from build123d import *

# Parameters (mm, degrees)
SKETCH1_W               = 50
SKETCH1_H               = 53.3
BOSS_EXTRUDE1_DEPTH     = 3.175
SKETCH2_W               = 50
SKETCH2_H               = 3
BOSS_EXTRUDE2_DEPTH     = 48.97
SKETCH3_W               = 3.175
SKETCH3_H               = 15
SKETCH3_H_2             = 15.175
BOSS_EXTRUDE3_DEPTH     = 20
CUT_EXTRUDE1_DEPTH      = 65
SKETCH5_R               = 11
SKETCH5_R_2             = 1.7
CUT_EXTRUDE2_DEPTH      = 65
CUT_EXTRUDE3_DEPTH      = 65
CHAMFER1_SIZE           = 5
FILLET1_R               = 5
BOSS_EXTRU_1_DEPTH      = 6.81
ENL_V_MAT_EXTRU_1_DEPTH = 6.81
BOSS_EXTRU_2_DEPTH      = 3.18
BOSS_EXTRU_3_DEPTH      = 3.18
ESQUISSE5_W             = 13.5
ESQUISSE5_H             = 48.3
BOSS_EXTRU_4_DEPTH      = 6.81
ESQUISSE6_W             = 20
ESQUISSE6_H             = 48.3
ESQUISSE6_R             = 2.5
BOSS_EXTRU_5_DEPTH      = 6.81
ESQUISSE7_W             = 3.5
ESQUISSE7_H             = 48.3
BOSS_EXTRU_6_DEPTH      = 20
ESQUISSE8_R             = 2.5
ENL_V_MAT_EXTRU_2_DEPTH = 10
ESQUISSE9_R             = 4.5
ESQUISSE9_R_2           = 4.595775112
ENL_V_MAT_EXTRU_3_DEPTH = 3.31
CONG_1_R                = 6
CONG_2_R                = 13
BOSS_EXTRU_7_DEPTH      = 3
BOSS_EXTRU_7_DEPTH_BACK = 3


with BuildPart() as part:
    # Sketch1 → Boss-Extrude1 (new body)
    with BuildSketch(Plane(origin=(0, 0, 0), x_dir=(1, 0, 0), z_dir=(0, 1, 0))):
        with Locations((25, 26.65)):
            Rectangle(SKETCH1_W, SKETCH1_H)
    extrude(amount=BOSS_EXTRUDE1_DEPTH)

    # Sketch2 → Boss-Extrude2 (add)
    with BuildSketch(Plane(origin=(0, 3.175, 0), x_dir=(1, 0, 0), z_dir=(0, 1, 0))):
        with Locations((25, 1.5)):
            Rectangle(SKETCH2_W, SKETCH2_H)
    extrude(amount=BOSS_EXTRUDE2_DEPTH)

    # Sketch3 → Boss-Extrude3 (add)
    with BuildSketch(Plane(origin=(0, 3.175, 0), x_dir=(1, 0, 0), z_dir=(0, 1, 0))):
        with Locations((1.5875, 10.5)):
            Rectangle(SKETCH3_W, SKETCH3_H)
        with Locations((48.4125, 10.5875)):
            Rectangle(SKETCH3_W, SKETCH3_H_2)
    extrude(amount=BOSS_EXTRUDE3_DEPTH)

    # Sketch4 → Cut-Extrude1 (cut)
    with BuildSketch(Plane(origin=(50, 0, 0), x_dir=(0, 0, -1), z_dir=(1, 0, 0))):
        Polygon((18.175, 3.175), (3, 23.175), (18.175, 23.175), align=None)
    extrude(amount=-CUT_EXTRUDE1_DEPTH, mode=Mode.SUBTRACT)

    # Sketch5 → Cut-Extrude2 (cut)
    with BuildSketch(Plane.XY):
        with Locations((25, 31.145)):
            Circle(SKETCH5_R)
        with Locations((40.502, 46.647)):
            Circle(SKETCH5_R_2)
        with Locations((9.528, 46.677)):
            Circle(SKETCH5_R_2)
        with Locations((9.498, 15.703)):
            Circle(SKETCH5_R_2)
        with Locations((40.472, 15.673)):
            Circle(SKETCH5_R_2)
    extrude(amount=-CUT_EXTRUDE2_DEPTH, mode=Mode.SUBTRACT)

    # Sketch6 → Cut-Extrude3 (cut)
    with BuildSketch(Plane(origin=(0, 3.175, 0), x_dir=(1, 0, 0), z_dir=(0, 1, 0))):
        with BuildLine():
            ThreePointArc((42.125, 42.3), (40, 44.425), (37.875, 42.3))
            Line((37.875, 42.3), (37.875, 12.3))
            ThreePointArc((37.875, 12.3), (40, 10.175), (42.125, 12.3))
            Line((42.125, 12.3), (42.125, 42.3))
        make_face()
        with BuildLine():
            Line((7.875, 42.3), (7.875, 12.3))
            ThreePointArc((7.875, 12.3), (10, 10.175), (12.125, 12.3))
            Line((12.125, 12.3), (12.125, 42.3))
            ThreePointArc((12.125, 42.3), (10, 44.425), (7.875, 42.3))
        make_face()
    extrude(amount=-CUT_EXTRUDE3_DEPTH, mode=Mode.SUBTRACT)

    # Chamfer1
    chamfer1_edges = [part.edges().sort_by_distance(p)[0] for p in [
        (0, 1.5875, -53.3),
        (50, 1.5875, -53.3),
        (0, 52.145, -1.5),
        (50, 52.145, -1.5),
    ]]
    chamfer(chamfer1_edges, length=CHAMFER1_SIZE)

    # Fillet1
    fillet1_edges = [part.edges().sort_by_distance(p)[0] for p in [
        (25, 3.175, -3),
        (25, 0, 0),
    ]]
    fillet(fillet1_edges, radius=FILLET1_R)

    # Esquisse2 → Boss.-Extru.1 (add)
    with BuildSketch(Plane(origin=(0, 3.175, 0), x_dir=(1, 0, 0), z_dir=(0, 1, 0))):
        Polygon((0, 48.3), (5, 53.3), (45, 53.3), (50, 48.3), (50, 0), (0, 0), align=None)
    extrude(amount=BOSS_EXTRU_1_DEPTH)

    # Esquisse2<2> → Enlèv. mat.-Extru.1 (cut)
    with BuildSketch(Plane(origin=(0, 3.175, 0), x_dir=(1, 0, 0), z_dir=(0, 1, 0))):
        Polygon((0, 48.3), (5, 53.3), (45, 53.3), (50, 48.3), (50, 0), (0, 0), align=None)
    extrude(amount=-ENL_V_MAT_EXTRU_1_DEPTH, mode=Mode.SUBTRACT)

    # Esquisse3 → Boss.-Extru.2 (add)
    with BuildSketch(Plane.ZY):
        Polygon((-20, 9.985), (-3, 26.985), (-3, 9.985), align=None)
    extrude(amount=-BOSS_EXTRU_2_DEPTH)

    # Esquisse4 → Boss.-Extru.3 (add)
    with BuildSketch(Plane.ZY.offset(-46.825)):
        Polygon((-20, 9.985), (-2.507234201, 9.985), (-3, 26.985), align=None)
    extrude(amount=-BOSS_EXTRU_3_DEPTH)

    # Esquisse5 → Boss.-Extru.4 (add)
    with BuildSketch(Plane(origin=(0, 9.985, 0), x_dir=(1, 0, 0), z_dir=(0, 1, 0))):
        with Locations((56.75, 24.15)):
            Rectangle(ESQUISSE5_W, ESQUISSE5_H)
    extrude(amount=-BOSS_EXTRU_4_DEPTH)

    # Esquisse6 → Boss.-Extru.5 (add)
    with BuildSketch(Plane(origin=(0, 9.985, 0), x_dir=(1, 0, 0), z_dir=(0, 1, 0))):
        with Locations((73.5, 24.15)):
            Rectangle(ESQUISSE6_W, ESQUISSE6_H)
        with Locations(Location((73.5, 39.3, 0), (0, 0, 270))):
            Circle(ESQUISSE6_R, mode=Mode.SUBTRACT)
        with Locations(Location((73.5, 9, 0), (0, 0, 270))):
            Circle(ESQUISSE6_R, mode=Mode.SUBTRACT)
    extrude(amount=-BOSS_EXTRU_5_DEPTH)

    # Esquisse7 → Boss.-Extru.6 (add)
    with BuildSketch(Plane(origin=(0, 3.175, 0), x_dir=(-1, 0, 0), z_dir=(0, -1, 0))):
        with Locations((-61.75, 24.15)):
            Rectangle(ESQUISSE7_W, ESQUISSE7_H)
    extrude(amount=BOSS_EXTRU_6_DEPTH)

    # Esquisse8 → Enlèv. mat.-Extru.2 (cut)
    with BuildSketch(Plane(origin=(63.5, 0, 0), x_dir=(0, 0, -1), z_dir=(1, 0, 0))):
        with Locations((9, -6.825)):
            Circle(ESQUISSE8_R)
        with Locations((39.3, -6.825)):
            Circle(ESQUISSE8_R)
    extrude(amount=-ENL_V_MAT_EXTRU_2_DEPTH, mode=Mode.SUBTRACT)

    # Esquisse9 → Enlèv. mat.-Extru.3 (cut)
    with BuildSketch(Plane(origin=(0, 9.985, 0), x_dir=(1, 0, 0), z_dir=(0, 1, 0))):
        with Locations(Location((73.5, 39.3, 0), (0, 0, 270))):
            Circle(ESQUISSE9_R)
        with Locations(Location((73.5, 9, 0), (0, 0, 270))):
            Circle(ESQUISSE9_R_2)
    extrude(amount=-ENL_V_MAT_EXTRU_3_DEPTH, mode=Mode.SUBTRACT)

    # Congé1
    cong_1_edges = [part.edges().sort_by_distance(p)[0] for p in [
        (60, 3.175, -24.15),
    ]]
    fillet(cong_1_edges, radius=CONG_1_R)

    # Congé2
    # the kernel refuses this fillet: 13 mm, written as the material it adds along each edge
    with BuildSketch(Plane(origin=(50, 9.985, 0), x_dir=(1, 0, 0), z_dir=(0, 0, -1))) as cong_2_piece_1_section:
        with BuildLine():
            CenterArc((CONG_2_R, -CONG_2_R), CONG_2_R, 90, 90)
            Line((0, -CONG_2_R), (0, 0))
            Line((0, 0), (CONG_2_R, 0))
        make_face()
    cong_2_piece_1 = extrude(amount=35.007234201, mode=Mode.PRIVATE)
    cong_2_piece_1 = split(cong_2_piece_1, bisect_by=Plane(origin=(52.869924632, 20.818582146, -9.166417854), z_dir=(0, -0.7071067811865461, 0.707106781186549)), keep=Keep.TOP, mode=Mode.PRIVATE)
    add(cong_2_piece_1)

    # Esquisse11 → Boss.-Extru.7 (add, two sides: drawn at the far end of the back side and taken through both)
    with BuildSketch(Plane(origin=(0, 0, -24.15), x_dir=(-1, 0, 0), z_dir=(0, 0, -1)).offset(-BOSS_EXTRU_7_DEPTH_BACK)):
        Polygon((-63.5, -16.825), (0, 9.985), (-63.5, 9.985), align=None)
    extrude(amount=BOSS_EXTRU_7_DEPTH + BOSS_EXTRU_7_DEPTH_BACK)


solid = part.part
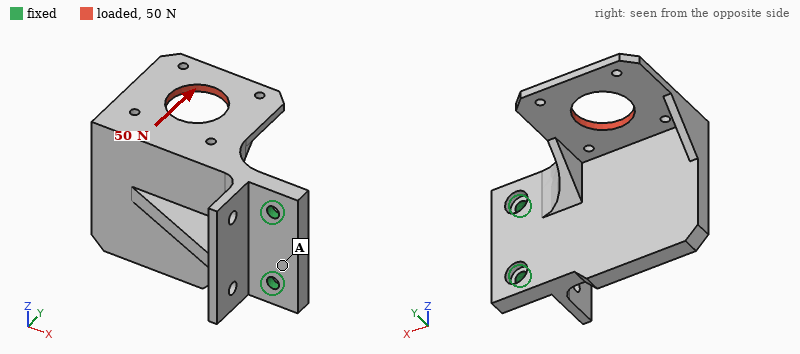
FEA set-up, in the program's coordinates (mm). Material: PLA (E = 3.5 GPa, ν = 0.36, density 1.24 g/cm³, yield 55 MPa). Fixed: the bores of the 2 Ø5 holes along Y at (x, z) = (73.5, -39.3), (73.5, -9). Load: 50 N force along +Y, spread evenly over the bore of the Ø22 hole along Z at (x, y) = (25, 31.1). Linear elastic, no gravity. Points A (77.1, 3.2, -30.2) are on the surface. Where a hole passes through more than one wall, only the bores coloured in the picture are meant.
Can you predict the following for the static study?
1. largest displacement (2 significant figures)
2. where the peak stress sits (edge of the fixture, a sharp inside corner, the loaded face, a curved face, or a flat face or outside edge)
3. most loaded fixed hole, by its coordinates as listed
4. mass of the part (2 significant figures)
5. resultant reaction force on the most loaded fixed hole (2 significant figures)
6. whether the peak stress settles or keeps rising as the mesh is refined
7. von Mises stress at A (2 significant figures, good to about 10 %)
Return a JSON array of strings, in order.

["1.2 mm", "edge of the fixture", "(73.5, -9)", "51 g", "59 N", "keeps rising", "2.1 MPa"]
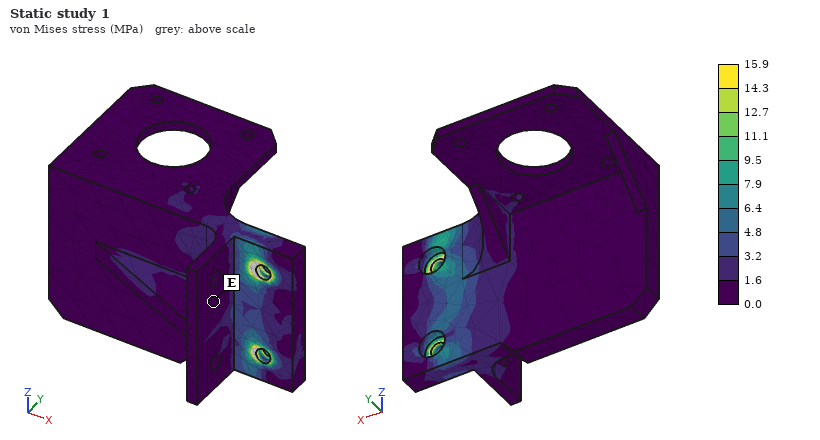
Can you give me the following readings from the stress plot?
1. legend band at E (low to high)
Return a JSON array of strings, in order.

["0.0 to 1.6 MPa"]
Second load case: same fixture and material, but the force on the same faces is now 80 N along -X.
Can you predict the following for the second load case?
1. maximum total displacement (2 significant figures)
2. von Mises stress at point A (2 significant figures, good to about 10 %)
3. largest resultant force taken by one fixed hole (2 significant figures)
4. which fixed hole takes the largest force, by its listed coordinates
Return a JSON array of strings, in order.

["1.2 mm", "1.7 MPa", "96 N", "(73.5, -9)"]
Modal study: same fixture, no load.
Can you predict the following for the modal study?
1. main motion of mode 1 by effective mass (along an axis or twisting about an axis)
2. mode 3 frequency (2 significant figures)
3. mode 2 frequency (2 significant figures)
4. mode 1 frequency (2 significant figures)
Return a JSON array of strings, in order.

["along Y", "950 Hz", "550 Hz", "240 Hz"]
